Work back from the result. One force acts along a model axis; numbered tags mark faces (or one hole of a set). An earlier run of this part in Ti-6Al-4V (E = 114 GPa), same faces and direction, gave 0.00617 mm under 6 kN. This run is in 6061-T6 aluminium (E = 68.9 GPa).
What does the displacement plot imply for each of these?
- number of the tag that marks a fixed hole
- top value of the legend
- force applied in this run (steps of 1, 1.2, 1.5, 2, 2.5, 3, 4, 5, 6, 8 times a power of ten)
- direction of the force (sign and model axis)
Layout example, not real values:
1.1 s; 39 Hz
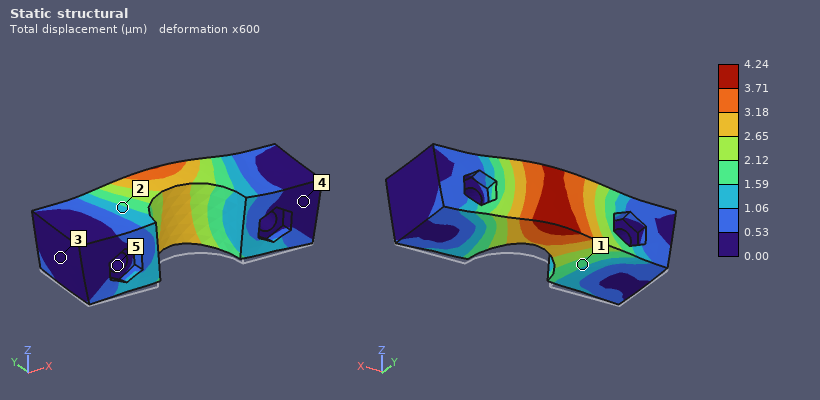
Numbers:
5; 4.24 µm; 2.5 kN; +Z
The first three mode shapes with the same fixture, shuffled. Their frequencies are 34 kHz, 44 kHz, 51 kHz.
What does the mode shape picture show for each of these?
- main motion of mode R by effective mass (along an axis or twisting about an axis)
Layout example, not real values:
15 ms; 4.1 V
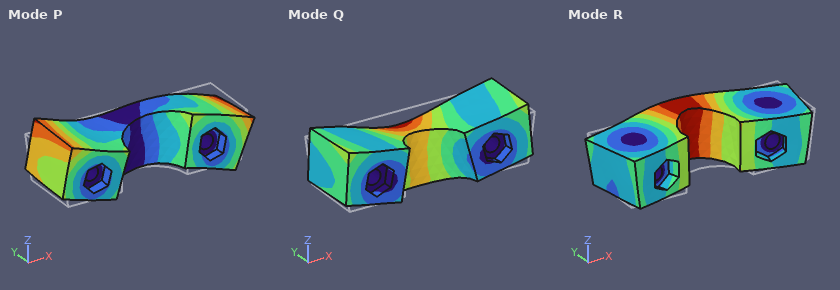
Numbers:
along Y
